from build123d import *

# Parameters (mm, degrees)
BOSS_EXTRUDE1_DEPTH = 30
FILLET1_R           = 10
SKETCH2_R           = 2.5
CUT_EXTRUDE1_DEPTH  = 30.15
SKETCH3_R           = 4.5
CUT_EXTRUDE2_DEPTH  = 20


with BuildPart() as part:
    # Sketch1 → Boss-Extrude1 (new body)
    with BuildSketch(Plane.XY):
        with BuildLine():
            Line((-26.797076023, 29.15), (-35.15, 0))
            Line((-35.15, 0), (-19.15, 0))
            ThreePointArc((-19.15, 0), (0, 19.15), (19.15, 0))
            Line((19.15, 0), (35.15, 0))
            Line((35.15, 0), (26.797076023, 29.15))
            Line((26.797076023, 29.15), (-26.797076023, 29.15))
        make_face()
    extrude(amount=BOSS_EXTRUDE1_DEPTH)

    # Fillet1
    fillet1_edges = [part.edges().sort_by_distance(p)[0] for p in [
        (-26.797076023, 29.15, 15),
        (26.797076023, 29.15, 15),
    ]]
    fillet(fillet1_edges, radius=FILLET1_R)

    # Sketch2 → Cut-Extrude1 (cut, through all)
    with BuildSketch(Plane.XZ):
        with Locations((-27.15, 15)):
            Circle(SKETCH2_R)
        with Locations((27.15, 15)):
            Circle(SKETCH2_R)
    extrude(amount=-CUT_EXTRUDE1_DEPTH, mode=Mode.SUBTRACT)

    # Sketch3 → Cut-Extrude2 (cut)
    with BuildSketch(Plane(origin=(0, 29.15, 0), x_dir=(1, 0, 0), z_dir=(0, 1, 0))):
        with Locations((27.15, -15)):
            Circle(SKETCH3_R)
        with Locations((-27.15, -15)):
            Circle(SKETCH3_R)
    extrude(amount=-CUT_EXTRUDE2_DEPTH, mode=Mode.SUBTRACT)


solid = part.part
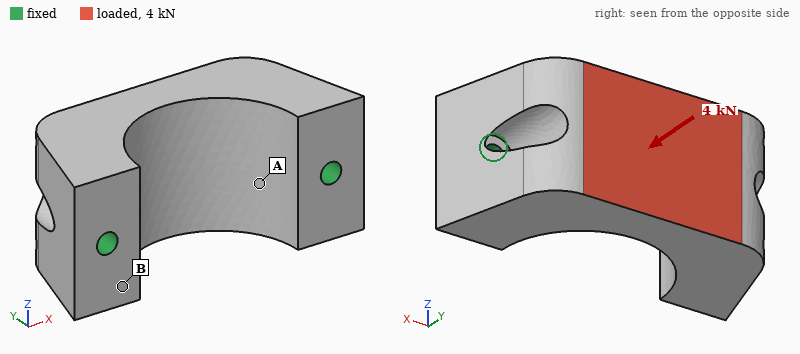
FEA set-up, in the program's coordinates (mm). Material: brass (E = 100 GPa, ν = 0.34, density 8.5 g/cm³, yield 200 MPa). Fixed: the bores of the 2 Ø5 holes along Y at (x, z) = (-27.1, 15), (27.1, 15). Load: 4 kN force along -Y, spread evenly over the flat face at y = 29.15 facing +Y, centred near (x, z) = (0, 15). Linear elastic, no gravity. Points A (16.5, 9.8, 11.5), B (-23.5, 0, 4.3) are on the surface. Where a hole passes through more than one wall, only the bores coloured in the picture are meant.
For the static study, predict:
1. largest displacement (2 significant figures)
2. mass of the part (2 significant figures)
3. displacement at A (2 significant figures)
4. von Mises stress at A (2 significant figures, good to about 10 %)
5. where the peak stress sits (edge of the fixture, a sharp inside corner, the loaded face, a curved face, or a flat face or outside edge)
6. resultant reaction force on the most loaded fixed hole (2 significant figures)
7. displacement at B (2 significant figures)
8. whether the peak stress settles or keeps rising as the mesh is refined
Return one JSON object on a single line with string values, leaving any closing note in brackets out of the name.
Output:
{"largest displacement": "6.0 µm", "mass of the part": "290 g", "displacement at A": "2.6 µm", "von Mises stress at A": "17 MPa", "where the peak stress sits": "edge of the fixture", "resultant reaction force on the most loaded fixed hole": "2.4 kN", "displacement at B": "2.3 µm", "whether the peak stress settles or keeps rising as the mesh is refined": "keeps rising"}
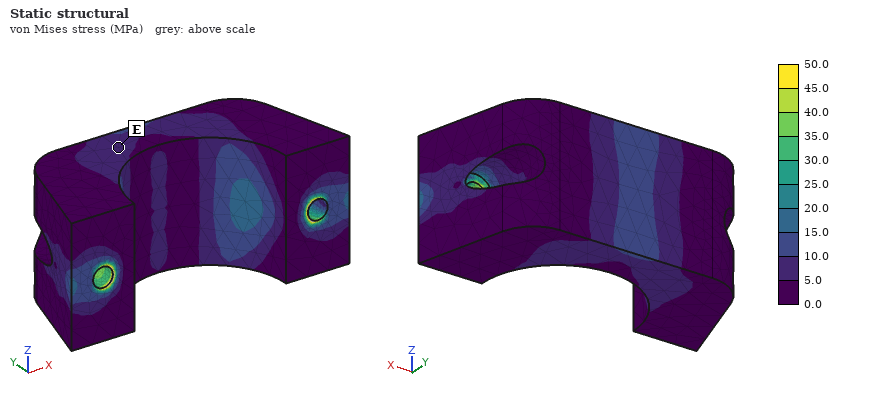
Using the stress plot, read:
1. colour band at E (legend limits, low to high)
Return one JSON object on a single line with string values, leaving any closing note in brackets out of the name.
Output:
{"colour band at E": "5.0 to 10.0 MPa"}
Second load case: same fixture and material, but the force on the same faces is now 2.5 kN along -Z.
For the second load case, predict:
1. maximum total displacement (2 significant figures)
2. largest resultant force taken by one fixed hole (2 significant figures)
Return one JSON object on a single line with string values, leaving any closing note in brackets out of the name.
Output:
{"maximum total displacement": "36 µm", "largest resultant force taken by one fixed hole": "1.3 kN"}
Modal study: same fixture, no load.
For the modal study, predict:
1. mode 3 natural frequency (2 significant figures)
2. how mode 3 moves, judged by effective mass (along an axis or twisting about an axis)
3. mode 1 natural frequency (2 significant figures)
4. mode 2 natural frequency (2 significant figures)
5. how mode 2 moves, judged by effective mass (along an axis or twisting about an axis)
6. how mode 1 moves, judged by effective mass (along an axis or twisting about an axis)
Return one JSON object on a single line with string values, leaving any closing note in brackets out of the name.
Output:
{"mode 3 natural frequency": "9100 Hz", "how mode 3 moves, judged by effective mass": "along X", "mode 1 natural frequency": "4100 Hz", "mode 2 natural frequency": "8600 Hz", "how mode 2 moves, judged by effective mass": "twisting about Y", "how mode 1 moves, judged by effective mass": "along Z"}
